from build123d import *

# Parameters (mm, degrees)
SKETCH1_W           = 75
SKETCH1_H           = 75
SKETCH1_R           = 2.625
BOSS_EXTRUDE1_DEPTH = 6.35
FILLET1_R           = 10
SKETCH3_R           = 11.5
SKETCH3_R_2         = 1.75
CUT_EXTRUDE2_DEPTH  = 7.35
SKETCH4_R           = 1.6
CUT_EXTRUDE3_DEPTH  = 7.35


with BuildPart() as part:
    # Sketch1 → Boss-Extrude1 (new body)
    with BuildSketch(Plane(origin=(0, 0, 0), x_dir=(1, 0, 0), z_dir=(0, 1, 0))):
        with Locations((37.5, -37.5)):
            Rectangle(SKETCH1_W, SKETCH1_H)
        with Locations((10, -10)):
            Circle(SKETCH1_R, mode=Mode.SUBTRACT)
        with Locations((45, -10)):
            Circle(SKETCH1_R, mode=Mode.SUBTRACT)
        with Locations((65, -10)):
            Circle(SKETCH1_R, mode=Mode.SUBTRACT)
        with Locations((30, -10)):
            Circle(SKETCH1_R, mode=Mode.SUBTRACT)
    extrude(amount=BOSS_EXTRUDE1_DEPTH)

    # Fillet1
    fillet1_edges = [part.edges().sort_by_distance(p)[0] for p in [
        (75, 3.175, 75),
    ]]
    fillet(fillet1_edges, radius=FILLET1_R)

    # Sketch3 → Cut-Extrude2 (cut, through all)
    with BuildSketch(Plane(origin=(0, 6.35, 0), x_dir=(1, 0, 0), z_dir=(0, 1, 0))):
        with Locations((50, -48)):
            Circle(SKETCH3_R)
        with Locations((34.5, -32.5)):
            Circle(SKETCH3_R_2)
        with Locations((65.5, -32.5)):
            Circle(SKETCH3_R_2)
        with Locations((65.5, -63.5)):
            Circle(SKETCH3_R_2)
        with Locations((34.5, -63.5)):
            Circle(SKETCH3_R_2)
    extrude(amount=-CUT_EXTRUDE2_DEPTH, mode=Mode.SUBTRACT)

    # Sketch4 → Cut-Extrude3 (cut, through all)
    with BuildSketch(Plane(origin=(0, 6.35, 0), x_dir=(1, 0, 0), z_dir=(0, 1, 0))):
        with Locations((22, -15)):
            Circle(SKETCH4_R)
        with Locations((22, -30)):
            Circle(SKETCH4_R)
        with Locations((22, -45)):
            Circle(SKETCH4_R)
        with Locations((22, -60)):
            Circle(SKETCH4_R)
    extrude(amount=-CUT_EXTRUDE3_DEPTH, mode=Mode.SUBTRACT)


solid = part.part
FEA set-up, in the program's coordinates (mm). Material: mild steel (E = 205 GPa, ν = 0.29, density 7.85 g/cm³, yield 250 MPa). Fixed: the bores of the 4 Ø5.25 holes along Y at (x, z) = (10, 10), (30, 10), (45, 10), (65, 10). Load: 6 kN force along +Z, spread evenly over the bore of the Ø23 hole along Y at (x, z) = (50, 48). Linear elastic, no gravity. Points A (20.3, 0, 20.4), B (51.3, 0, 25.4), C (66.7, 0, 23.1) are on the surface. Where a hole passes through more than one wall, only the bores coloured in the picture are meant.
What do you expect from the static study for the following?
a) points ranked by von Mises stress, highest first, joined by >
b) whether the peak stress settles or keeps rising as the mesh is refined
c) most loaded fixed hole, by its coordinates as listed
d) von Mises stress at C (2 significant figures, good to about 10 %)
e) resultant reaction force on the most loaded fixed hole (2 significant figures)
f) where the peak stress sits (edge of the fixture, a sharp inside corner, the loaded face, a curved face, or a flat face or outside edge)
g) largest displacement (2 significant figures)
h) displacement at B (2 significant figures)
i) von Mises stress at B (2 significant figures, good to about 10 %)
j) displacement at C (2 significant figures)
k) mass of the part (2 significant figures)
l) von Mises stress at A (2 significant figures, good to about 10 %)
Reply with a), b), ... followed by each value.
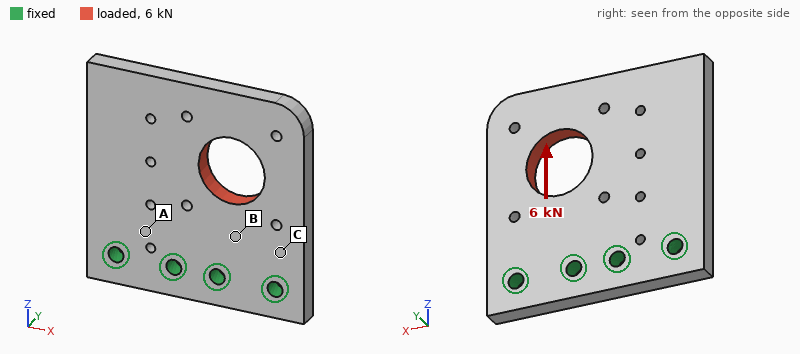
a) C > B > A
b) keeps rising
c) (65, 10)
d) 23 MPa
e) 3.0 kN
f) edge of the fixture
g) 7.7 µm
h) 1.4 µm
i) 15 MPa
j) 2.0 µm
k) 250 g
l) 6.8 MPa
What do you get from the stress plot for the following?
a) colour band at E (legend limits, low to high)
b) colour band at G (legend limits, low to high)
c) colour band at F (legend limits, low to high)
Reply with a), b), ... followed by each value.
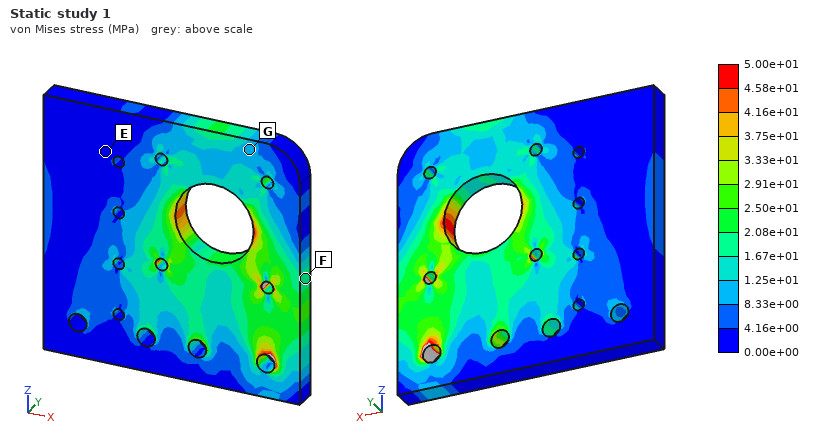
a) 0.00e+00 to 4.16e+00 MPa
b) 8.33e+00 to 1.25e+01 MPa
c) 1.67e+01 to 2.08e+01 MPa
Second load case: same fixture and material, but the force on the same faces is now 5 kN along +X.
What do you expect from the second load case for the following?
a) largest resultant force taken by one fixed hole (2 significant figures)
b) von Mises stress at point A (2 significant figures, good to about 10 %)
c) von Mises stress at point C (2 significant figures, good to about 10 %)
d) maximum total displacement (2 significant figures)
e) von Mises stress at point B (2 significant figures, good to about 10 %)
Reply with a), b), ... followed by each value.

a) 3.3 kN
b) 24 MPa
c) 19 MPa
d) 16 µm
e) 34 MPa
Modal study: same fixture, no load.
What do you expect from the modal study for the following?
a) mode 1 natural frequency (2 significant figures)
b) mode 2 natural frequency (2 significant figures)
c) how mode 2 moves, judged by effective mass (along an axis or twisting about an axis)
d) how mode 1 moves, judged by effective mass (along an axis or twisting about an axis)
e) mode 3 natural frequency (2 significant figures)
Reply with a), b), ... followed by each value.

a) 1300 Hz
b) 2600 Hz
c) twisting about Z
d) along Y
e) 6500 Hz
